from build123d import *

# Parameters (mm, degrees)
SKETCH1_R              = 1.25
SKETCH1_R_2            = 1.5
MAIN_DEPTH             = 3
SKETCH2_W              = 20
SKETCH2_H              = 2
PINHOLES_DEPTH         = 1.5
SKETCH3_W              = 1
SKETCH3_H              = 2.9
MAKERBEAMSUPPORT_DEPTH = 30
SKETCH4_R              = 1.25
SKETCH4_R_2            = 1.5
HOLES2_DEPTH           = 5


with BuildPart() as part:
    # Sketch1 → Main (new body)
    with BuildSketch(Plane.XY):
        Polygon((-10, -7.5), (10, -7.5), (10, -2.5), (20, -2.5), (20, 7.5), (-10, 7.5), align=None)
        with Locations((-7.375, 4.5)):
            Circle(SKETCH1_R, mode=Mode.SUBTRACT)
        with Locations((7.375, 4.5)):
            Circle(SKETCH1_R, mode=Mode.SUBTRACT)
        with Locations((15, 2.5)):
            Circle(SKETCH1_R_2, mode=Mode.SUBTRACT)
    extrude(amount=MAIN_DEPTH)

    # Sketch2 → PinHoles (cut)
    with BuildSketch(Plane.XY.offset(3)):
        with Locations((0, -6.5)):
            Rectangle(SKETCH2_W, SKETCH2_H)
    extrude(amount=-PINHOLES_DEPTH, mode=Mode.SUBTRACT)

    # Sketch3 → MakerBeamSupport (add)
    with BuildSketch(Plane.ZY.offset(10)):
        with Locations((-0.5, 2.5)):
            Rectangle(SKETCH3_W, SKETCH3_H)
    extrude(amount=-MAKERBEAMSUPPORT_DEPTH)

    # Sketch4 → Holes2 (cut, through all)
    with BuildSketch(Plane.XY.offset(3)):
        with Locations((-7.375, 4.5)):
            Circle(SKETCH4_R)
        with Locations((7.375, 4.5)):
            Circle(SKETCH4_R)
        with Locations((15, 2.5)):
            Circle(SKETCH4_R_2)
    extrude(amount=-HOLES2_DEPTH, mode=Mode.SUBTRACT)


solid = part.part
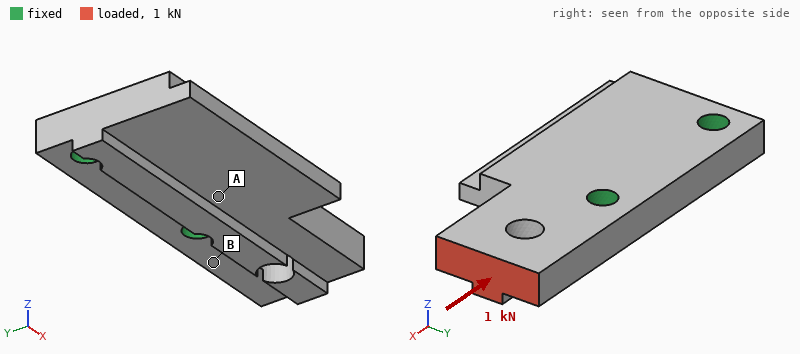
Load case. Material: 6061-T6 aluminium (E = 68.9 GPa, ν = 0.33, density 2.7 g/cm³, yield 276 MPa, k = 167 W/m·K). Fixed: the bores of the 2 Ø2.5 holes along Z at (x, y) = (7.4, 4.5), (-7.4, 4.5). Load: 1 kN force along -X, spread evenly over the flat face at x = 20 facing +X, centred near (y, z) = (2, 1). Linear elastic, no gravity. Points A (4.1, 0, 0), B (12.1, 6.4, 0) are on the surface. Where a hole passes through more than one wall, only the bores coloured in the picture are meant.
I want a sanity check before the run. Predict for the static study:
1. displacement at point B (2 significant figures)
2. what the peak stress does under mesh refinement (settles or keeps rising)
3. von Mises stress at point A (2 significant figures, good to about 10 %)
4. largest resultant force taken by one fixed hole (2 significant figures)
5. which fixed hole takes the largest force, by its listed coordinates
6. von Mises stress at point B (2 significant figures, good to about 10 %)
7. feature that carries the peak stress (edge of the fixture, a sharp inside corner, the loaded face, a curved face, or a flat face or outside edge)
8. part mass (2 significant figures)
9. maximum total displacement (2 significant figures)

2.5 µm
keeps rising
15 MPa
850 N
(7.4, 4.5)
47 MPa
a sharp inside corner
3.2 g
13 µm
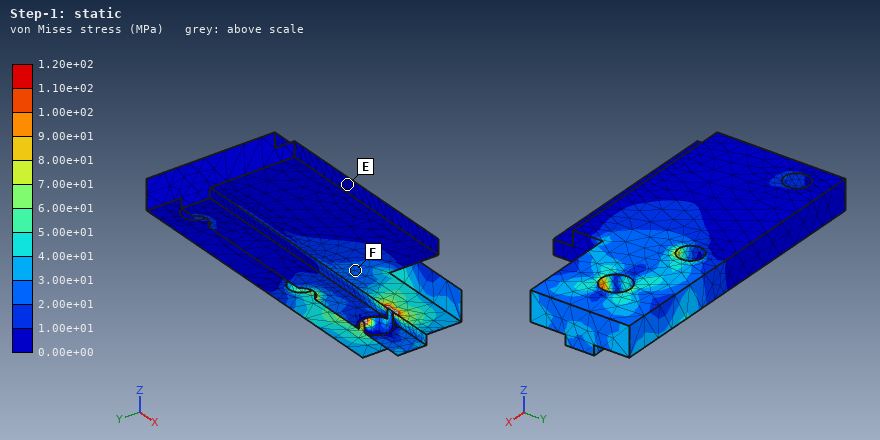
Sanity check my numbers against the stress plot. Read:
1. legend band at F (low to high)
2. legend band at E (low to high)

2.00e+01 to 3.00e+01 MPa
0.00e+00 to 1.00e+01 MPa
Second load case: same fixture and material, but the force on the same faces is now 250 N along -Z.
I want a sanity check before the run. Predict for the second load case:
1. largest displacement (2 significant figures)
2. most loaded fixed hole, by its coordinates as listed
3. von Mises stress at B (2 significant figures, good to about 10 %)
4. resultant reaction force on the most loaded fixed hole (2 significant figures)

97 µm
(7.4, 4.5)
120 MPa
300 N
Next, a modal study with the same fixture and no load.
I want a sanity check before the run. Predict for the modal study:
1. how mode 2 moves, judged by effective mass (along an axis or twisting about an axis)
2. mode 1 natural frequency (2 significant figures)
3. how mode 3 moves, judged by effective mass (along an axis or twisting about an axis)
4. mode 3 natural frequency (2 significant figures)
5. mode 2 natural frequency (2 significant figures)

along Z
17 kHz
along Y
30 kHz
21 kHz
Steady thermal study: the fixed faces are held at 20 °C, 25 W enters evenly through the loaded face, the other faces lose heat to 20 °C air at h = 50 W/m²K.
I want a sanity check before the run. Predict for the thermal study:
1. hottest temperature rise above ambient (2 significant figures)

68 K
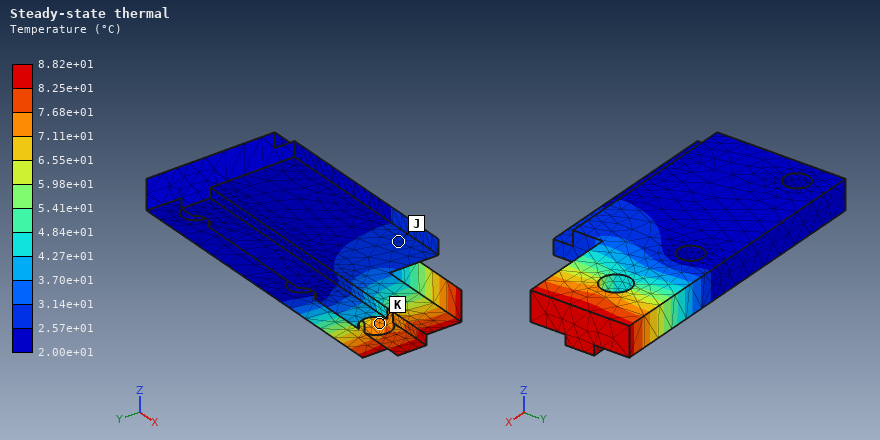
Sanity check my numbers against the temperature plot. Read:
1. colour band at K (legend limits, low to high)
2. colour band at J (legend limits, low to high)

7.11e+01 to 7.68e+01 °C
2.57e+01 to 3.14e+01 °C
